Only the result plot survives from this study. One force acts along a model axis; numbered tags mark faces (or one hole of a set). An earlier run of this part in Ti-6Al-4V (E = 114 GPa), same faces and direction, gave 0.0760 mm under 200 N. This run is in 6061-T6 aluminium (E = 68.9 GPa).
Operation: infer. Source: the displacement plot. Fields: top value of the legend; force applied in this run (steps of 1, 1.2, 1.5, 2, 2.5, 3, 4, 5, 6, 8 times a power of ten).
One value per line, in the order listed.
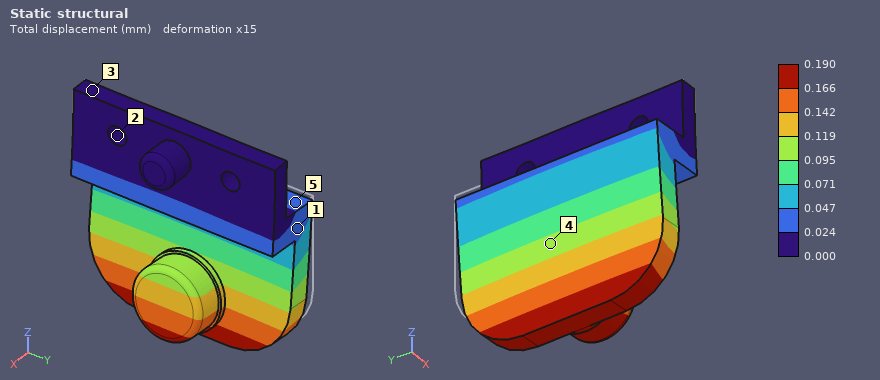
0.190 mm
300 N
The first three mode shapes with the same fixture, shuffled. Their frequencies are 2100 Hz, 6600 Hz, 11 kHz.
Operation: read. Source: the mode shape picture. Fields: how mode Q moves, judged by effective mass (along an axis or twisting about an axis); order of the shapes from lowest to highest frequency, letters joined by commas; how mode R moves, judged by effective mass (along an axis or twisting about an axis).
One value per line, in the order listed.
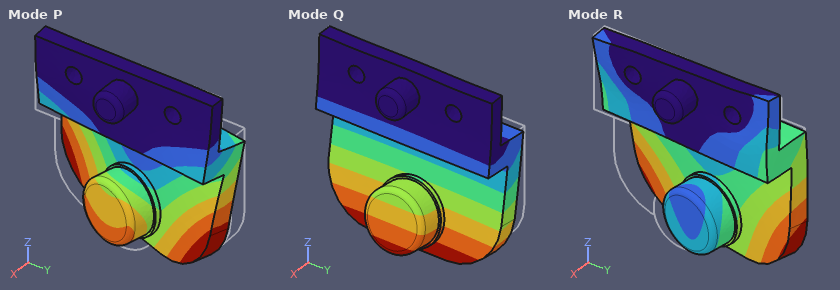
along X
Q, P, R
along Y
